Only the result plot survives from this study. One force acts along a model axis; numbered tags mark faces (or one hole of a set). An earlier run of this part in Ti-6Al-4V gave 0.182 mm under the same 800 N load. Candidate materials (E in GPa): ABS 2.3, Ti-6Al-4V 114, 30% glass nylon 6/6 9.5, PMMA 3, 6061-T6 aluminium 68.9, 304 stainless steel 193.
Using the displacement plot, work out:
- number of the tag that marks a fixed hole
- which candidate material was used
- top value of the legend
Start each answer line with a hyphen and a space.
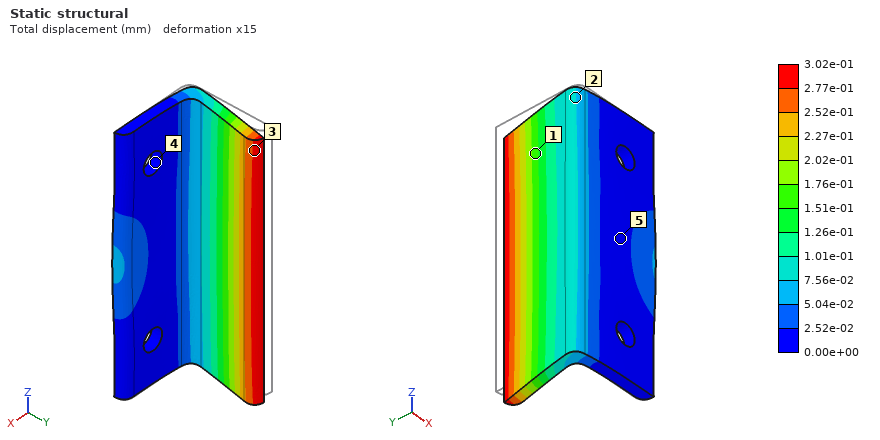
- 4
- 6061-T6 aluminium
- 3.02e-01 mm
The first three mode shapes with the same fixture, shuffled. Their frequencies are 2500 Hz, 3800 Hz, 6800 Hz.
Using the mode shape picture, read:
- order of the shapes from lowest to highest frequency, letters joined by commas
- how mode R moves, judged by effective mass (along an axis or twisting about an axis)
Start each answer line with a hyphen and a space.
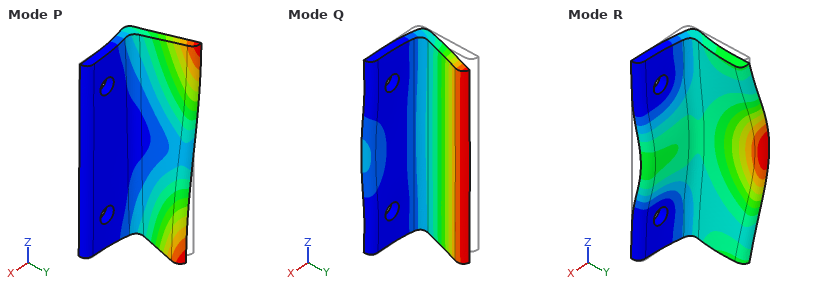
- Q, P, R
- along Y
